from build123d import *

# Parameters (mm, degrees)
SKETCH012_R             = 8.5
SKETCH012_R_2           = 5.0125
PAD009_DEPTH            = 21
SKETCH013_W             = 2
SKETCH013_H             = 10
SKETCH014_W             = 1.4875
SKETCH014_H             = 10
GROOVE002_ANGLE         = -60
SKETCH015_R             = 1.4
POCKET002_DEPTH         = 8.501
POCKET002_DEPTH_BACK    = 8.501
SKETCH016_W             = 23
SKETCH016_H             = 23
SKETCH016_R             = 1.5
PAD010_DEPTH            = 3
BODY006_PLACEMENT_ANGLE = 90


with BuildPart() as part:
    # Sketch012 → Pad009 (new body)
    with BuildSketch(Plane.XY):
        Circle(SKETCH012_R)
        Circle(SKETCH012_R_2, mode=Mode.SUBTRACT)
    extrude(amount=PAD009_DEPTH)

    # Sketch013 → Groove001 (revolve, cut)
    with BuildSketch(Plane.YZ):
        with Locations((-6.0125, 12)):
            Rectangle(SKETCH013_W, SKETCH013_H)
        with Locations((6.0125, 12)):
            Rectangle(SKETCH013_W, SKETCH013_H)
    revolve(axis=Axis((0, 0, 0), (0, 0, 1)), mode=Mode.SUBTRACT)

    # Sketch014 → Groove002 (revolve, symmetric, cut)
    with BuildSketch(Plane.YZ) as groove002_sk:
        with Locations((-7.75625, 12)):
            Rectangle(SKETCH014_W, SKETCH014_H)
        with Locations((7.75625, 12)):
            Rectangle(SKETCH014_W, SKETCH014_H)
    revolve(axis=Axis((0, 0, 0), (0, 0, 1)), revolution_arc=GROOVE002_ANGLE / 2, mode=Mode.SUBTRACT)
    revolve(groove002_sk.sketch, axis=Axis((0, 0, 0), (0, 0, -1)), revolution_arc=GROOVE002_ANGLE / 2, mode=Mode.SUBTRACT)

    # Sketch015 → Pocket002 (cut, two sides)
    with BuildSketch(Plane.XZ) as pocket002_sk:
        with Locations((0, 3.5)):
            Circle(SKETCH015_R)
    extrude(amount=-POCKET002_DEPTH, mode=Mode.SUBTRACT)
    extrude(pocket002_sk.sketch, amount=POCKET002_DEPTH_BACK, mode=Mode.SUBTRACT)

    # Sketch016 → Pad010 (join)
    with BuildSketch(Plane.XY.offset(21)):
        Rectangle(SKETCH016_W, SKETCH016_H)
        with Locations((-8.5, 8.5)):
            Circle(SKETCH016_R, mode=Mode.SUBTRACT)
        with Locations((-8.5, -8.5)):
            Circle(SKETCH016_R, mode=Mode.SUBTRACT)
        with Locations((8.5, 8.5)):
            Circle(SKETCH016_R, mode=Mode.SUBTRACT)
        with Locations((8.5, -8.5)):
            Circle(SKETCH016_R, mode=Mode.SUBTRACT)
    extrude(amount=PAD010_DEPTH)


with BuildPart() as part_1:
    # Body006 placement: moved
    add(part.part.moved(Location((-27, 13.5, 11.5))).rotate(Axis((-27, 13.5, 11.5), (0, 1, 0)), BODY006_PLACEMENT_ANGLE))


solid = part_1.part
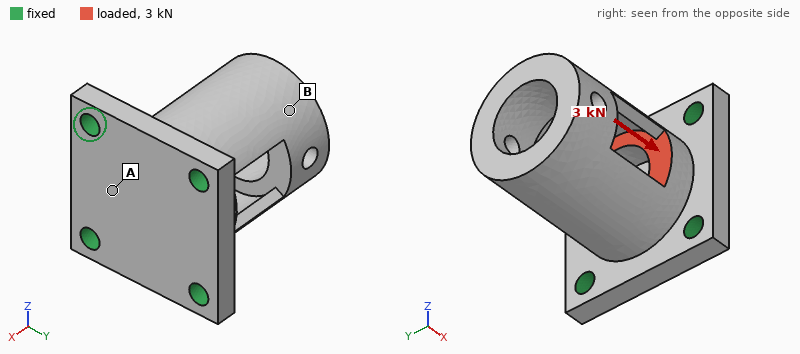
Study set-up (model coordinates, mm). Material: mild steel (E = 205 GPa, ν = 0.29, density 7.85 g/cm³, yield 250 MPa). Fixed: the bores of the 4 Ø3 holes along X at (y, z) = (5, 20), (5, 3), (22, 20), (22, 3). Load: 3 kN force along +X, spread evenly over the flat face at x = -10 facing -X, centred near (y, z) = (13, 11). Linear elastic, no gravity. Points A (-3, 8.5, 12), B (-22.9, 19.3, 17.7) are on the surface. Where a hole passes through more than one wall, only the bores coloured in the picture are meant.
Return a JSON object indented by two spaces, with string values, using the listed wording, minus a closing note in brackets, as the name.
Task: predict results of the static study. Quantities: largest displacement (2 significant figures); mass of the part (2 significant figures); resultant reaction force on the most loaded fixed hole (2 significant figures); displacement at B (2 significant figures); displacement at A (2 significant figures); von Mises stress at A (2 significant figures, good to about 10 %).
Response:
{
  "largest displacement": "4.3 µm",
  "mass of the part": "28 g",
  "resultant reaction force on the most loaded fixed hole": "790 N",
  "displacement at B": "3.1 µm",
  "displacement at A": "4.0 µm",
  "von Mises stress at A": "31 MPa"
}
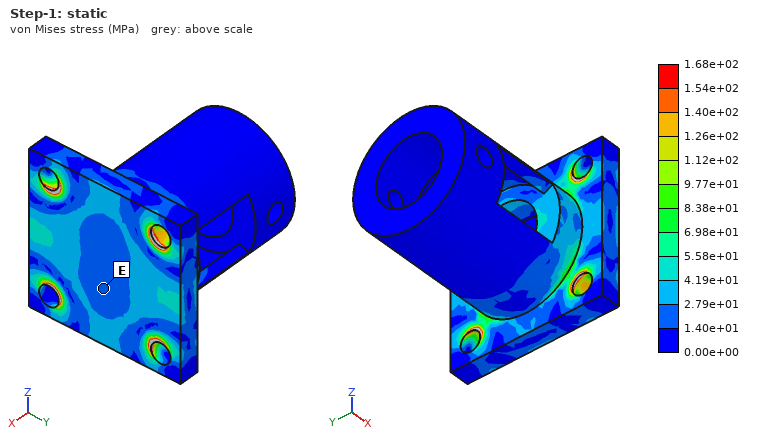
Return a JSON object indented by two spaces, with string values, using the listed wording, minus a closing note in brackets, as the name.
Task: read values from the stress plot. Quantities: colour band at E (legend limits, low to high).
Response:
{
  "colour band at E": "1.40e+01 to 2.79e+01 MPa"
}
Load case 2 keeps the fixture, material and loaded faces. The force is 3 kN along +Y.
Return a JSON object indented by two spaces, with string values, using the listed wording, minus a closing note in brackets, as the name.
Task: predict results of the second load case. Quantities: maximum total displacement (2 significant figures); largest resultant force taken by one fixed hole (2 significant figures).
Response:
{
  "maximum total displacement": "9.3 µm",
  "largest resultant force taken by one fixed hole": "950 N"
}
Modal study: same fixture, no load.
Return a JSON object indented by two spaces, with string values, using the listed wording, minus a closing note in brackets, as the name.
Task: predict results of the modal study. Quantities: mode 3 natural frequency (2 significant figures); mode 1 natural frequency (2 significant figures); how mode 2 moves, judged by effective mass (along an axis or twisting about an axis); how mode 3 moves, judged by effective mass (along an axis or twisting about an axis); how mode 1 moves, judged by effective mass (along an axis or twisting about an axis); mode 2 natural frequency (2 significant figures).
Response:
{
  "mode 3 natural frequency": "21 kHz",
  "mode 1 natural frequency": "8500 Hz",
  "how mode 2 moves, judged by effective mass": "along Y",
  "how mode 3 moves, judged by effective mass": "twisting about X",
  "how mode 1 moves, judged by effective mass": "along Z",
  "mode 2 natural frequency": "11 kHz"
}
